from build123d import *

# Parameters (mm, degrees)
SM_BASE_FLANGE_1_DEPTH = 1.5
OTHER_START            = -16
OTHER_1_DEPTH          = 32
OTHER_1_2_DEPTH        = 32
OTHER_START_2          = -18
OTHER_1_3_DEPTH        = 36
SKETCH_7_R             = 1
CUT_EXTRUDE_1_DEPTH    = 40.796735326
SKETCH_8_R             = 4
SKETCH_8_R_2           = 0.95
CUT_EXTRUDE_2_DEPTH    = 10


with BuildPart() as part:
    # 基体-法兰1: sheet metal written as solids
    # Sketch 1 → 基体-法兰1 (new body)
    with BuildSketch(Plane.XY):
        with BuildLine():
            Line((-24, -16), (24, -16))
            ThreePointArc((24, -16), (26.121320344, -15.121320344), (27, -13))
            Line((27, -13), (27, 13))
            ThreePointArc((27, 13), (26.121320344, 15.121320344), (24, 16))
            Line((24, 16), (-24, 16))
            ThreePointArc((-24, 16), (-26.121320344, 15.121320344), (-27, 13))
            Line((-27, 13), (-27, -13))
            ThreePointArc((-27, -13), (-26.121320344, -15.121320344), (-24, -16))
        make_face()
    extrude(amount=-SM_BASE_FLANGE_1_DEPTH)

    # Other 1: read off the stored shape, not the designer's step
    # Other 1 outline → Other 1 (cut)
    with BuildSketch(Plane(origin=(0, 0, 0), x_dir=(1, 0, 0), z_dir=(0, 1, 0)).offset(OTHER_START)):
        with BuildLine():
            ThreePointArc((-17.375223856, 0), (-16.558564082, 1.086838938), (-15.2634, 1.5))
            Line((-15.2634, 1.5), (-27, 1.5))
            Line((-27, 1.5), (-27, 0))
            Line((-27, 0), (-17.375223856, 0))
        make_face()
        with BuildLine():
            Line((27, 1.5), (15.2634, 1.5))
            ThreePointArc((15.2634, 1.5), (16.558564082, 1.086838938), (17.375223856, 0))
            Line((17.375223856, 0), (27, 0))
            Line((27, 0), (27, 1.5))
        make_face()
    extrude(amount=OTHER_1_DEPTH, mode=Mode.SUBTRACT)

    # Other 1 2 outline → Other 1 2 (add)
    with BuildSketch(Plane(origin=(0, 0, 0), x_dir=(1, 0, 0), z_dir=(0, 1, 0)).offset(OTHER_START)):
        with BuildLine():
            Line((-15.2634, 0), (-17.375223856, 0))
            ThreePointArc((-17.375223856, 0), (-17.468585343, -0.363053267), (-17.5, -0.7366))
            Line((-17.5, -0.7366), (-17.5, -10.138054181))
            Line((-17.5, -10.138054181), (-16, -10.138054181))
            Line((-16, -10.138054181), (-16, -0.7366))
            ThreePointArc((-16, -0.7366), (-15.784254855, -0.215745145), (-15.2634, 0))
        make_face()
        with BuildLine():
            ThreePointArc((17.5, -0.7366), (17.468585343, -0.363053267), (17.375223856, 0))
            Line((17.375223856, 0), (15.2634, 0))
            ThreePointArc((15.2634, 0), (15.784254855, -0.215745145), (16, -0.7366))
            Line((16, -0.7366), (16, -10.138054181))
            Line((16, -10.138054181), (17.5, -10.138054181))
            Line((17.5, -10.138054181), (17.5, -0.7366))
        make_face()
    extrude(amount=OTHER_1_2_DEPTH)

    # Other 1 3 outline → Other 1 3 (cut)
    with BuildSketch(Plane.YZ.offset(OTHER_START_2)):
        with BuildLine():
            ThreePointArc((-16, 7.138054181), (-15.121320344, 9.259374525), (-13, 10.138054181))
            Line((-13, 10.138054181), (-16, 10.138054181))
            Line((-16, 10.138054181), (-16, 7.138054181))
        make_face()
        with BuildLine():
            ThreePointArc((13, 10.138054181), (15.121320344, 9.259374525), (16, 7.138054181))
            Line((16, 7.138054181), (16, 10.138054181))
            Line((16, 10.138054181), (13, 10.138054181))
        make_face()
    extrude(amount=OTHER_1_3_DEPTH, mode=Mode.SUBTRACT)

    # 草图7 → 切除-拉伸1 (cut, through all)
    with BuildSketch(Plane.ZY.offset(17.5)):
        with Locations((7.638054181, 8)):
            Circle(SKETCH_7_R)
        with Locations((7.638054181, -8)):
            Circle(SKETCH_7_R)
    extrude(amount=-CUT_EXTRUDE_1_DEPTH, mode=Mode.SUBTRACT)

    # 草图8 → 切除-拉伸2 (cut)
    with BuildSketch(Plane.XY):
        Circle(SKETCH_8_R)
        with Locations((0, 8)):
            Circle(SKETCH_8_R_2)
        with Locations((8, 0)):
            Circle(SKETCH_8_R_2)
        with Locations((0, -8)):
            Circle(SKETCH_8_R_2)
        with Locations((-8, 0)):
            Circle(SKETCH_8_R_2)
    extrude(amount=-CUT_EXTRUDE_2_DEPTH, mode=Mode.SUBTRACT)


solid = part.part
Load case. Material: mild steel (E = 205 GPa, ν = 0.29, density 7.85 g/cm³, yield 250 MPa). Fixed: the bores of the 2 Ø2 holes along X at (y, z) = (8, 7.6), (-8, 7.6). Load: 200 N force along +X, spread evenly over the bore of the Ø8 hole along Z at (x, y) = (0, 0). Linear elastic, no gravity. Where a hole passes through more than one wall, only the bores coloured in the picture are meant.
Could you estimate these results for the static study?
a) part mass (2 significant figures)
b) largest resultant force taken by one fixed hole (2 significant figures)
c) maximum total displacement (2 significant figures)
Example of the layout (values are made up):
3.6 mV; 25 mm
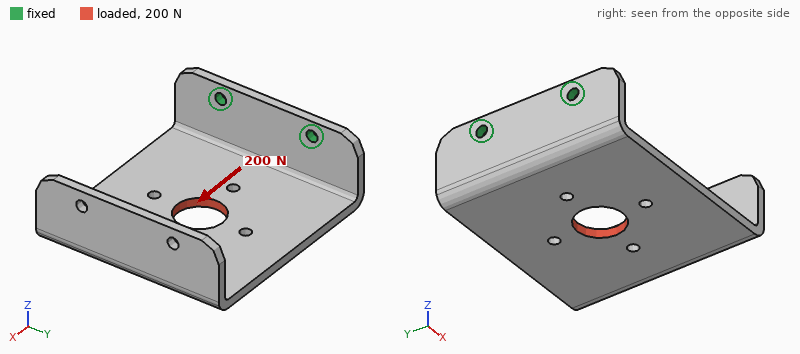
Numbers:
19 g; 100 N; 0.16 mm
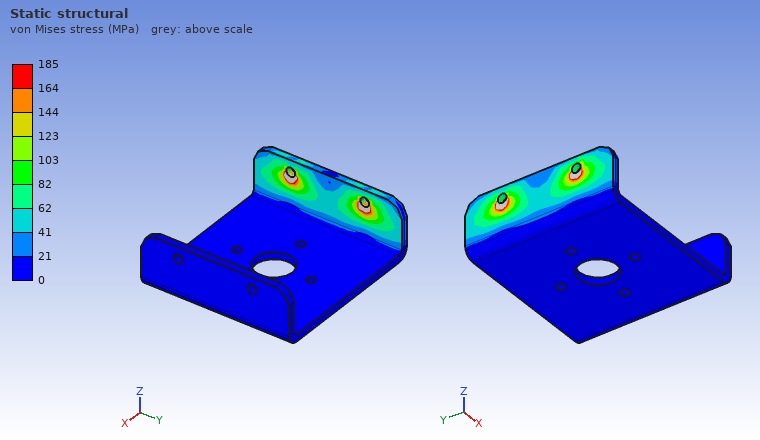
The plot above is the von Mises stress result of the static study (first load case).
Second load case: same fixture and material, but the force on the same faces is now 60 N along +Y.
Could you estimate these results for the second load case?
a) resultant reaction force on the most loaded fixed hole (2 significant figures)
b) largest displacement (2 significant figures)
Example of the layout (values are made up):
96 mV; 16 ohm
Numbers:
68 N; 42 µm
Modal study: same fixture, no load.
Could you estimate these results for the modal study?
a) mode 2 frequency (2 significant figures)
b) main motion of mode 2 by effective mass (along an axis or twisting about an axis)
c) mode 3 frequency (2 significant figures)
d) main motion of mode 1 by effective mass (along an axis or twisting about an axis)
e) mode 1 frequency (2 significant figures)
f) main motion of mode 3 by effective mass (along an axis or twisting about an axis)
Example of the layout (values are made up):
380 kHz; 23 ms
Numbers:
1300 Hz; along Y; 2300 Hz; along Z; 540 Hz; along Y
